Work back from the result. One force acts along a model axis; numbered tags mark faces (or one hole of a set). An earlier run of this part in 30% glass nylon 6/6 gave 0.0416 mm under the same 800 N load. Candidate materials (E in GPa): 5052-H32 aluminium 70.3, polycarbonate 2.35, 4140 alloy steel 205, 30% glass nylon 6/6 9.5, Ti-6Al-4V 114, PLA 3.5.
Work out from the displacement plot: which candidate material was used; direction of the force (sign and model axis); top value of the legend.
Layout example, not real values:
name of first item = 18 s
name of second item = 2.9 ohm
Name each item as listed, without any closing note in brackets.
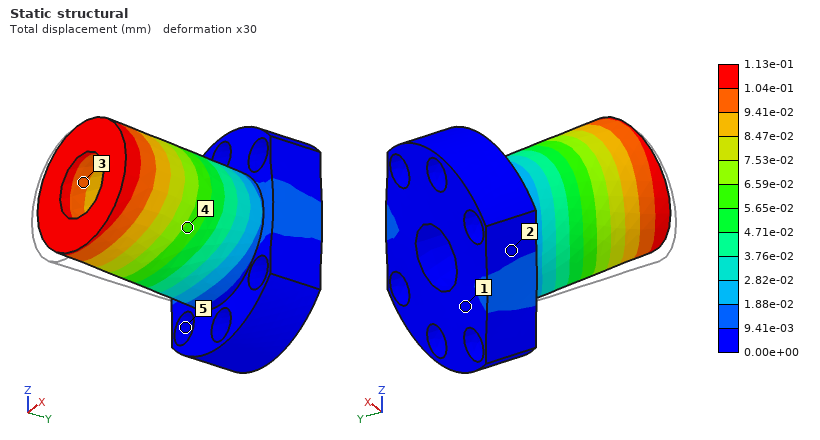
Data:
which candidate material was used = PLA
direction of the force = +X
top value of the legend = 1.13e-01 mm
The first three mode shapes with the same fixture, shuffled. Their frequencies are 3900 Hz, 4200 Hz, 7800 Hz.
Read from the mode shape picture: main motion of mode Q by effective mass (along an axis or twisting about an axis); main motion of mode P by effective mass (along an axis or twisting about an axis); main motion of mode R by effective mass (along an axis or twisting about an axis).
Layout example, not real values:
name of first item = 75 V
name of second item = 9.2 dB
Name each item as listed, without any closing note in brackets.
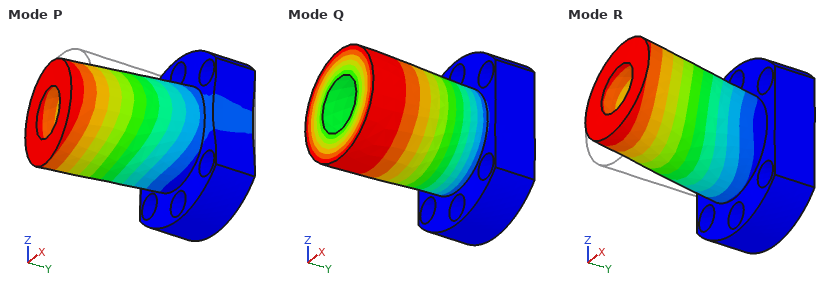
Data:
main motion of mode Q by effective mass = twisting about Y
main motion of mode P by effective mass = along X
main motion of mode R by effective mass = along Z
